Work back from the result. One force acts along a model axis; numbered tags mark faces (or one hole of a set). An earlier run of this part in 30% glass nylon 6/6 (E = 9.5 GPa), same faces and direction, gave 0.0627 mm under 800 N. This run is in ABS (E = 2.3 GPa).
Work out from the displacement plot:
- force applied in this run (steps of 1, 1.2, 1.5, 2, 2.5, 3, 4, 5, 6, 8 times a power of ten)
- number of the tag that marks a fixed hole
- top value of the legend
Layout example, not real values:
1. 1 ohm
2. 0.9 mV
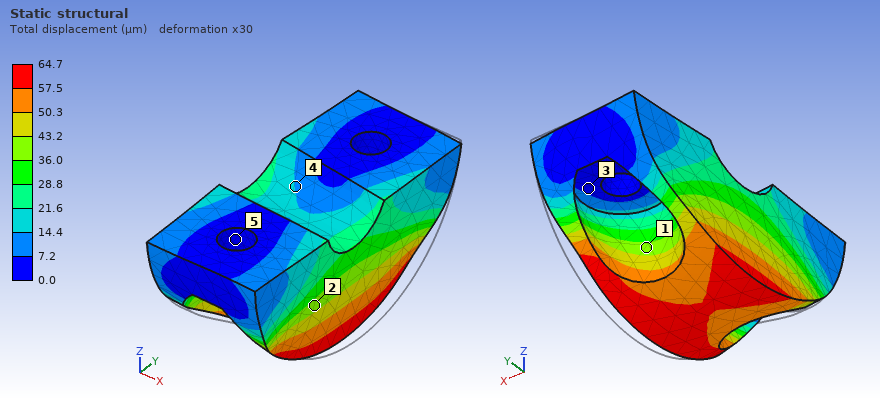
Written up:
1. 200 N
2. 5
3. 64.7 µm
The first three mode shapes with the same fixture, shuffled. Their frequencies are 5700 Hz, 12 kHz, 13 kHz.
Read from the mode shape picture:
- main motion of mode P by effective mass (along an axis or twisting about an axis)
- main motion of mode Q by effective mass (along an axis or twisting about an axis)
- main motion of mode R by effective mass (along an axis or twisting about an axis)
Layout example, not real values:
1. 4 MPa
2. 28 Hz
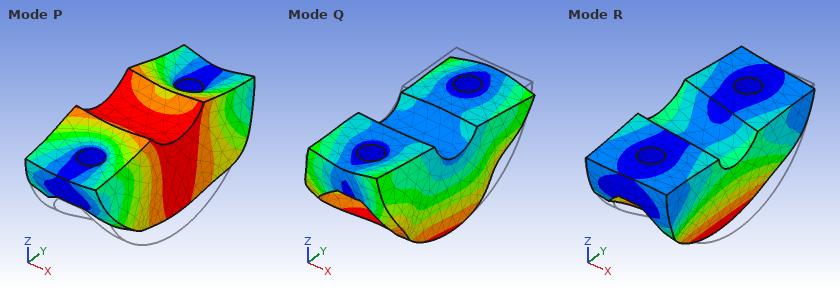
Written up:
1. along Z
2. along Y
3. along X
